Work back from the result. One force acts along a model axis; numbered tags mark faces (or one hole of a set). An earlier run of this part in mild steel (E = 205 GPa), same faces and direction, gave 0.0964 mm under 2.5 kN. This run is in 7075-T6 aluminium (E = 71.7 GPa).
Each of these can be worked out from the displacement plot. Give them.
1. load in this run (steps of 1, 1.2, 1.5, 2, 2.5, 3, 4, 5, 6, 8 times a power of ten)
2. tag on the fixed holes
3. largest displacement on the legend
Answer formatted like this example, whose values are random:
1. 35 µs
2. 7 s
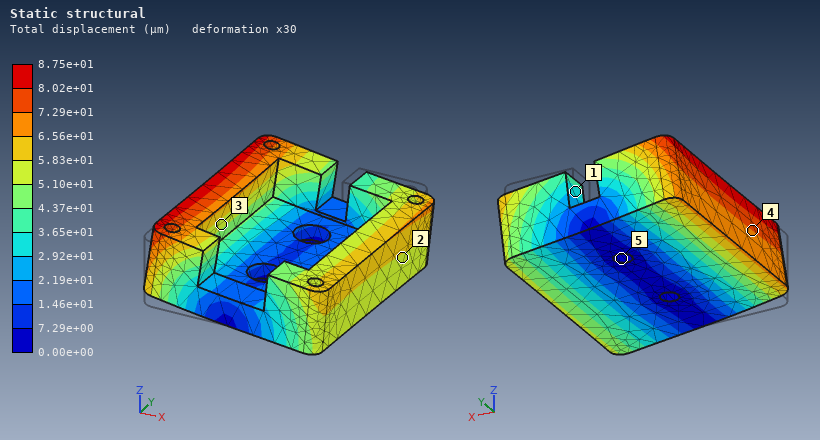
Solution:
1. 800 N
2. 5
3. 8.75e+01 µm
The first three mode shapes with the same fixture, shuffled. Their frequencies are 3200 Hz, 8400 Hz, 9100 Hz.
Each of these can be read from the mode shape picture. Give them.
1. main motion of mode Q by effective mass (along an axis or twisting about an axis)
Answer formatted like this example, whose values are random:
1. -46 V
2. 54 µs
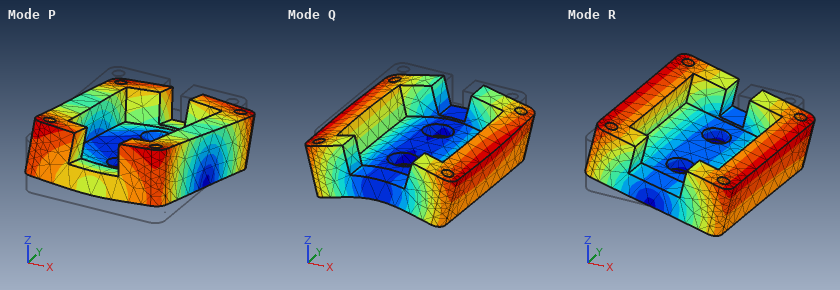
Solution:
1. along Z
